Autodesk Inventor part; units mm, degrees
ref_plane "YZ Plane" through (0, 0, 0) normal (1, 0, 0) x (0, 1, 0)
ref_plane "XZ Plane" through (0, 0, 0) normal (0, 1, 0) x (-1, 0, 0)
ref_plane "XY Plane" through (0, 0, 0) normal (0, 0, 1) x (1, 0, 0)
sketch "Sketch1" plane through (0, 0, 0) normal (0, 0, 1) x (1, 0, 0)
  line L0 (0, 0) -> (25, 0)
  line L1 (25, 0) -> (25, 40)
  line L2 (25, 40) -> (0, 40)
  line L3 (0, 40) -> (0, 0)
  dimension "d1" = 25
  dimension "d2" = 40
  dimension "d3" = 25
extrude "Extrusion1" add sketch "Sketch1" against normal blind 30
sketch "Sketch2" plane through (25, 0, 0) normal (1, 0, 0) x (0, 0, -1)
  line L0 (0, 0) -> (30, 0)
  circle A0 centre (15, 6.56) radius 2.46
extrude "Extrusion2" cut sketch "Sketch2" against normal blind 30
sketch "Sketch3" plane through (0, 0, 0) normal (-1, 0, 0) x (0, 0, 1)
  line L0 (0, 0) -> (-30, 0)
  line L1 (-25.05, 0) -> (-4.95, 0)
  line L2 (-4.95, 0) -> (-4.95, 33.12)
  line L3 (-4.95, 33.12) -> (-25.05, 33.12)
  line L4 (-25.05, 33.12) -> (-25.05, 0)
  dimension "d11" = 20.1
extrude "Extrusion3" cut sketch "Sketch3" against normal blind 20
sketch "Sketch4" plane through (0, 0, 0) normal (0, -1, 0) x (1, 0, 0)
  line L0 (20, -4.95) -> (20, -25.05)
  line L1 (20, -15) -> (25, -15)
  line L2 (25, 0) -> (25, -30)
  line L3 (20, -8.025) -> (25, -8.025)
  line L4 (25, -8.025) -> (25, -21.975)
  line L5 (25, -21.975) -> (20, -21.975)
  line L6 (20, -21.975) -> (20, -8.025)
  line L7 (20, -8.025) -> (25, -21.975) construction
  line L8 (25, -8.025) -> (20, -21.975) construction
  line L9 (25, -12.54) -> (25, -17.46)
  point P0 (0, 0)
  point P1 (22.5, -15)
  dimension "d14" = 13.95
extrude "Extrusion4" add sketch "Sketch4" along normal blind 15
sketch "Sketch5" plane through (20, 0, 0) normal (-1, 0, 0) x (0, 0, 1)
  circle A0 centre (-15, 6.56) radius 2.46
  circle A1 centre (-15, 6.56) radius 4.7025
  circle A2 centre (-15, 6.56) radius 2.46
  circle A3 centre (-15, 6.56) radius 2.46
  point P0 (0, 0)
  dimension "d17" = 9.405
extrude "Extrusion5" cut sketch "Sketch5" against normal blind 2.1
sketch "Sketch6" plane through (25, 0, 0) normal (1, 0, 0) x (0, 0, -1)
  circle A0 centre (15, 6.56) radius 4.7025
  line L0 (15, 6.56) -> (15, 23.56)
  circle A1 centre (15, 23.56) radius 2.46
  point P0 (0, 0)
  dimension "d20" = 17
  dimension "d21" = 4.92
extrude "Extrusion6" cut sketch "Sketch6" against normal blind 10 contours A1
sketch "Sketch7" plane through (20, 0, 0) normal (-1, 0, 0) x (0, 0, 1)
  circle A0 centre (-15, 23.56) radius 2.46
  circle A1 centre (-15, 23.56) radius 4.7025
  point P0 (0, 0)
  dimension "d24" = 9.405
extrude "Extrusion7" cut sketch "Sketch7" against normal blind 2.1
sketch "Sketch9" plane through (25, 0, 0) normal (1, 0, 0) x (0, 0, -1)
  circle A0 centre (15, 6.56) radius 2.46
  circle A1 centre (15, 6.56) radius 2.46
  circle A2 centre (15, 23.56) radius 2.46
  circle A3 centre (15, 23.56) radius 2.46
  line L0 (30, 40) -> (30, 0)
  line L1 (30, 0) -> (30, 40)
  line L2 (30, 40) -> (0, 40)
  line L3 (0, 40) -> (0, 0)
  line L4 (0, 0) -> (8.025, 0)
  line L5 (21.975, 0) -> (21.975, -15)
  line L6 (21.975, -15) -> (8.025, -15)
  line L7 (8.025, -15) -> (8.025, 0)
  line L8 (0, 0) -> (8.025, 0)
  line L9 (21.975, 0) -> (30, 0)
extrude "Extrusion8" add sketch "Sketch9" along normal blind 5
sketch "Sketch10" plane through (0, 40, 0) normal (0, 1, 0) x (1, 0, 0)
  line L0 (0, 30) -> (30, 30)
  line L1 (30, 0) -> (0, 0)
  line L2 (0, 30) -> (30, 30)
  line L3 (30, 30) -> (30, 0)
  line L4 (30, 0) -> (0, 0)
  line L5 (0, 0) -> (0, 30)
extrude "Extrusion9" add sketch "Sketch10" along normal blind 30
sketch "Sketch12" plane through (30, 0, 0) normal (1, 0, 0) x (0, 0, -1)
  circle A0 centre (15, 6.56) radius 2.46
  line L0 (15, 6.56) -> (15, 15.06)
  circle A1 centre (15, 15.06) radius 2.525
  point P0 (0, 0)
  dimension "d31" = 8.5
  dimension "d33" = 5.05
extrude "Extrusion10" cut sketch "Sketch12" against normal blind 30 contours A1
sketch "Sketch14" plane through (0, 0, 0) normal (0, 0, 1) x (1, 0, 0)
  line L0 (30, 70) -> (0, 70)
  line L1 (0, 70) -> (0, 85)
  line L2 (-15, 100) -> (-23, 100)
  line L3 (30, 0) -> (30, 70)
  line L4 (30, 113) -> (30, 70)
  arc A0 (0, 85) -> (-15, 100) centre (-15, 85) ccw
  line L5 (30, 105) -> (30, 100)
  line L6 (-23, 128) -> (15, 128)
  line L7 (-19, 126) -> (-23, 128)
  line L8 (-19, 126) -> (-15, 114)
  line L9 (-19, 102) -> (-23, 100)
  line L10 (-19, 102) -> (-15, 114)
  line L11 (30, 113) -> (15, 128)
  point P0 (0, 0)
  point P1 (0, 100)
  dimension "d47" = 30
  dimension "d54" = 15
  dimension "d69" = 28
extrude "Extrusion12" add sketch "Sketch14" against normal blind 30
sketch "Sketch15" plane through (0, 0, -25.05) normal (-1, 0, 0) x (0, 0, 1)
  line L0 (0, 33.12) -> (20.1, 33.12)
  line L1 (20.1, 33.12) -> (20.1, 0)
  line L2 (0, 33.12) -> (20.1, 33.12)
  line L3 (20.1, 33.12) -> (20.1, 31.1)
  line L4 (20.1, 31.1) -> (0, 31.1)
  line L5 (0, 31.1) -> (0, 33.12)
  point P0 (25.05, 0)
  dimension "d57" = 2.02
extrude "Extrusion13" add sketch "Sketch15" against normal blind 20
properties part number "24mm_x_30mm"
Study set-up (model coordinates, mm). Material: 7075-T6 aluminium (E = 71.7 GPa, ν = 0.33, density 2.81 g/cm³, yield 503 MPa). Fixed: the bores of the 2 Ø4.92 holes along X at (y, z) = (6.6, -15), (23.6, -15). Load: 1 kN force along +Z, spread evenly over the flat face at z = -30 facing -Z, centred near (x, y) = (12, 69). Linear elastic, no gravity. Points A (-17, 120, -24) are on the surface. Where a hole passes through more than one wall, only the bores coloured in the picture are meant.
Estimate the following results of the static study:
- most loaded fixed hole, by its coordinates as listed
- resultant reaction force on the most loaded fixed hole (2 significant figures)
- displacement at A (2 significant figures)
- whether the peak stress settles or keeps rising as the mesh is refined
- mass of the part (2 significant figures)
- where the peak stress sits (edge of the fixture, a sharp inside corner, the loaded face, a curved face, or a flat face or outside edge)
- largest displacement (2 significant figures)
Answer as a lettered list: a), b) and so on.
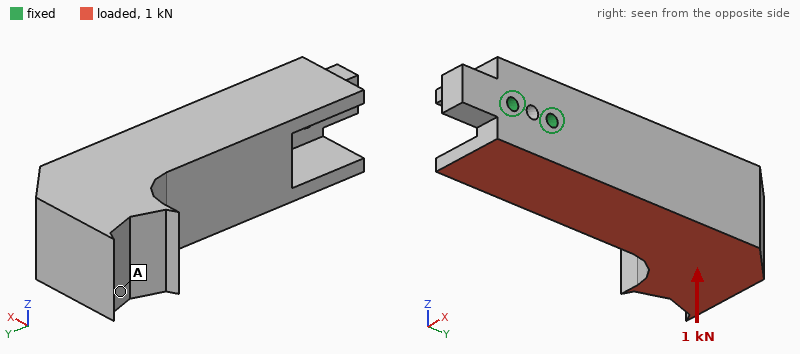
a) (23.6, -15)
b) 2.9 kN
c) 0.10 mm
d) keeps rising
e) 330 g
f) edge of the fixture
g) 0.11 mm
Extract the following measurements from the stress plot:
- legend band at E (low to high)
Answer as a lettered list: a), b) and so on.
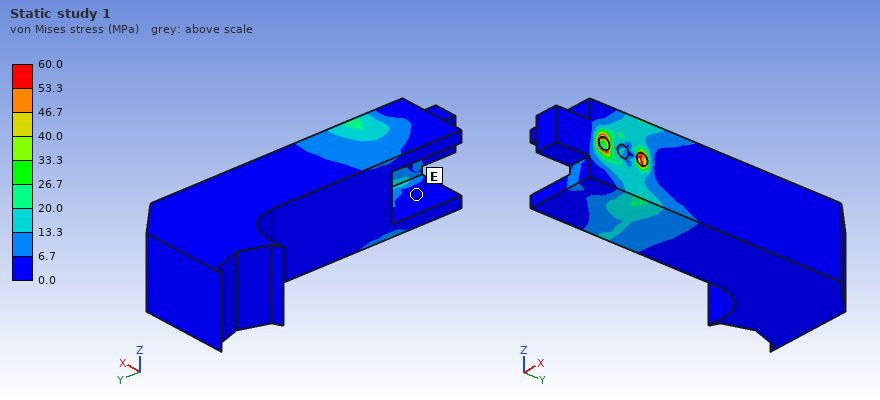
a) 0.0 to 6.7 MPa
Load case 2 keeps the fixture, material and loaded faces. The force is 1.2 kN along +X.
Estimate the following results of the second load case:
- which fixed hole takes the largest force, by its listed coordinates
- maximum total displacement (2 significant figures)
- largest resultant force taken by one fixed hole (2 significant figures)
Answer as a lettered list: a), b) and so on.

a) (23.6, -15)
b) 0.19 mm
c) 3.2 kN
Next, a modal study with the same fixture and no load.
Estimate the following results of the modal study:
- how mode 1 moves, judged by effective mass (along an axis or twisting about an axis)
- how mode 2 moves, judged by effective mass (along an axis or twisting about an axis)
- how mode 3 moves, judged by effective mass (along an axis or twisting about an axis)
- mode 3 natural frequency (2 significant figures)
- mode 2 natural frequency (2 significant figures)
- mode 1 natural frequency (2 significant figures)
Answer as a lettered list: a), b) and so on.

a) along X
b) along Z
c) twisting about Y
d) 2800 Hz
e) 1000 Hz
f) 860 Hz
